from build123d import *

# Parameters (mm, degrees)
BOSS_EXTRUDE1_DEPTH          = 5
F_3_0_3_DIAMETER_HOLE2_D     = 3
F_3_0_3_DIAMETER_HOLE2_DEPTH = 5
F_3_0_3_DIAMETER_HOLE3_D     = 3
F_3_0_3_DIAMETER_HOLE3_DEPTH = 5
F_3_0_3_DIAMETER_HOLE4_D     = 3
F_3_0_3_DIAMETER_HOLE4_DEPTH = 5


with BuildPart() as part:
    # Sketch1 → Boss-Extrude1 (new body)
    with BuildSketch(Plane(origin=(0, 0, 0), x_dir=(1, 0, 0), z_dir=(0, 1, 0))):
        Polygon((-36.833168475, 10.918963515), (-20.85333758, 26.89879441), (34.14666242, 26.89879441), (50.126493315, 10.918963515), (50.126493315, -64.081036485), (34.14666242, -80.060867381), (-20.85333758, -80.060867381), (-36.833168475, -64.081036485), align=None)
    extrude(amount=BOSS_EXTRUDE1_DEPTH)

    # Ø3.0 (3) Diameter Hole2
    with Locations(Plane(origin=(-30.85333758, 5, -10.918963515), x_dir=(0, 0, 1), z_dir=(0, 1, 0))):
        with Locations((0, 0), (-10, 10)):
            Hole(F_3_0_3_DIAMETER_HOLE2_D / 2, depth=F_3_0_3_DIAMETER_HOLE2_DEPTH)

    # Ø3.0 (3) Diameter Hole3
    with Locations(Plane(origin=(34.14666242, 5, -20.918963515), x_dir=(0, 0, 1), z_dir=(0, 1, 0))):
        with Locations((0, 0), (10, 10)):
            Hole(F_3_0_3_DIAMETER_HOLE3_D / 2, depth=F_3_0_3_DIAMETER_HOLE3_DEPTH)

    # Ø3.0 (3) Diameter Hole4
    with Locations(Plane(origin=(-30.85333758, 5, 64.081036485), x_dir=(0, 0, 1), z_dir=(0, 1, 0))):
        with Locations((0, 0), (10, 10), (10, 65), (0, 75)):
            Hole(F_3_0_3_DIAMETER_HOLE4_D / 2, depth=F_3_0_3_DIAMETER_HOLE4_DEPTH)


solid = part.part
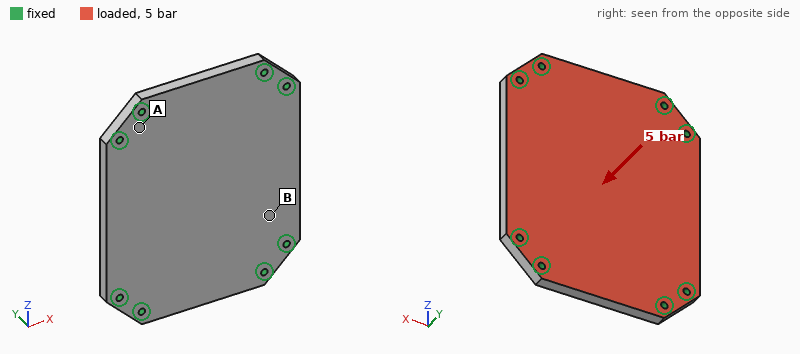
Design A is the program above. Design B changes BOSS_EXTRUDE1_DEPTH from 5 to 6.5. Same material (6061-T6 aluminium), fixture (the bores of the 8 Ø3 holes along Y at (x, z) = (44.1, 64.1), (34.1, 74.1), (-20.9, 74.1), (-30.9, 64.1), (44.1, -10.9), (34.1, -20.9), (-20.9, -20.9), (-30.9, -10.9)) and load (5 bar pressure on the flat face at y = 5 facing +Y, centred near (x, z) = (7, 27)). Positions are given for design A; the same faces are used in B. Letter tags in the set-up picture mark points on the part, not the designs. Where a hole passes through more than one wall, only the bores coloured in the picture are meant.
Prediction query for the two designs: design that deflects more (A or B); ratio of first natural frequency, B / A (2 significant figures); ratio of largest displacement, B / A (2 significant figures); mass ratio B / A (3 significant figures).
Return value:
A
1.3
0.48
1.30
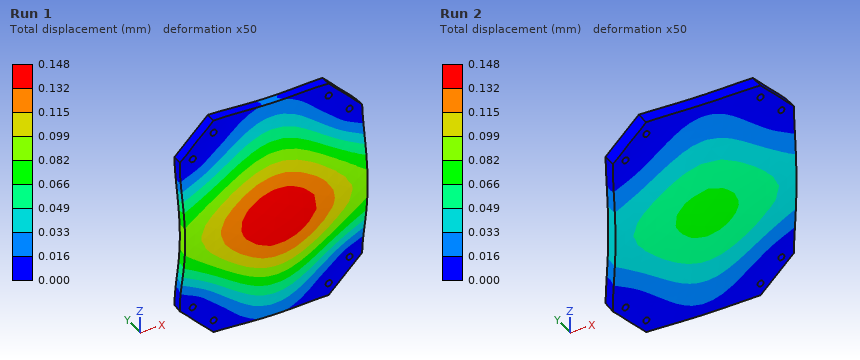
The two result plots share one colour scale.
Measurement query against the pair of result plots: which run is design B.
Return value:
Run 2
